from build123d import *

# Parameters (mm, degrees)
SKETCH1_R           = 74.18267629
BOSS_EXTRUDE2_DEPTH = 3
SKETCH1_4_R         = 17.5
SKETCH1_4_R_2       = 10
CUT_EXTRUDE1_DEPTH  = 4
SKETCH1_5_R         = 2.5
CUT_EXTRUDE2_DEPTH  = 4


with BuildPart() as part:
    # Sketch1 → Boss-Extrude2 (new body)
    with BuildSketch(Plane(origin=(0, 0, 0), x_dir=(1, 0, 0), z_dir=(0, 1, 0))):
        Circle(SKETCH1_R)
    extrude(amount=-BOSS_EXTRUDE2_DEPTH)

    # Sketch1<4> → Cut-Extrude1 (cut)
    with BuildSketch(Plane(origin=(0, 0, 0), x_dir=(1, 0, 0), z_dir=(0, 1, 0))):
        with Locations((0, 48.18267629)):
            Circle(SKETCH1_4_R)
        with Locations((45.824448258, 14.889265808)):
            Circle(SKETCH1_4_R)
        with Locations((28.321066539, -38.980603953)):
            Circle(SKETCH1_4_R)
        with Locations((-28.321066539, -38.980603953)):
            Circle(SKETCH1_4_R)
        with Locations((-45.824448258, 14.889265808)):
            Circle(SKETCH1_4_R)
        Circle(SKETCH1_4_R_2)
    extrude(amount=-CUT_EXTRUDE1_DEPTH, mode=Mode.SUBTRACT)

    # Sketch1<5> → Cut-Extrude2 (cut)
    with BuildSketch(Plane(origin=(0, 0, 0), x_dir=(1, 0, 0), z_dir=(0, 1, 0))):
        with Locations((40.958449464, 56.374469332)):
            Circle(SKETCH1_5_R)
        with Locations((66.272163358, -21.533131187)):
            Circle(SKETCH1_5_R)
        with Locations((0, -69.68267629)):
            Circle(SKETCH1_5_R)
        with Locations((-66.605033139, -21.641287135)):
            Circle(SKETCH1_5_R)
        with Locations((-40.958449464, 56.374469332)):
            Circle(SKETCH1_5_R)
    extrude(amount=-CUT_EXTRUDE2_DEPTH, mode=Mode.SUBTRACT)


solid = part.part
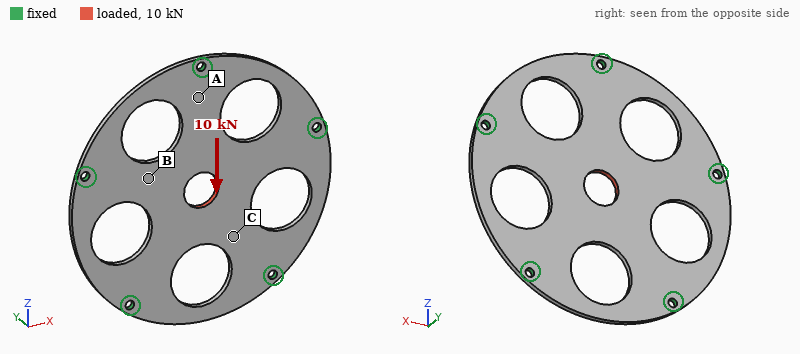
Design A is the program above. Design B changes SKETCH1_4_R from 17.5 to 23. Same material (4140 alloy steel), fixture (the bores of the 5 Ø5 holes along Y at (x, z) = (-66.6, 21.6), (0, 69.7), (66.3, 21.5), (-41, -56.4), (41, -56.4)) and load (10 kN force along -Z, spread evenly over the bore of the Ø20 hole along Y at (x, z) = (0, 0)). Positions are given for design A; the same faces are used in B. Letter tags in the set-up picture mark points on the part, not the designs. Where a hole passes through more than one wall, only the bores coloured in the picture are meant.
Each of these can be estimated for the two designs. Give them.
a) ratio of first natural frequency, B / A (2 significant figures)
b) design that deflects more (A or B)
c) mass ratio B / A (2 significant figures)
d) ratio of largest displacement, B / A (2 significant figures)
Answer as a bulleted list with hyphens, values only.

- 0.99
- B
- 0.71
- 1.5
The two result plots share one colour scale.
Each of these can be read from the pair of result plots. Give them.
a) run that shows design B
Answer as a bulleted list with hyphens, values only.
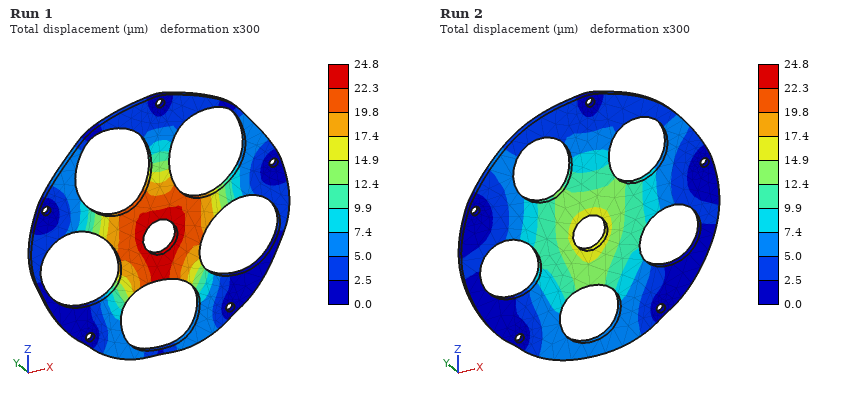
- Run 1
